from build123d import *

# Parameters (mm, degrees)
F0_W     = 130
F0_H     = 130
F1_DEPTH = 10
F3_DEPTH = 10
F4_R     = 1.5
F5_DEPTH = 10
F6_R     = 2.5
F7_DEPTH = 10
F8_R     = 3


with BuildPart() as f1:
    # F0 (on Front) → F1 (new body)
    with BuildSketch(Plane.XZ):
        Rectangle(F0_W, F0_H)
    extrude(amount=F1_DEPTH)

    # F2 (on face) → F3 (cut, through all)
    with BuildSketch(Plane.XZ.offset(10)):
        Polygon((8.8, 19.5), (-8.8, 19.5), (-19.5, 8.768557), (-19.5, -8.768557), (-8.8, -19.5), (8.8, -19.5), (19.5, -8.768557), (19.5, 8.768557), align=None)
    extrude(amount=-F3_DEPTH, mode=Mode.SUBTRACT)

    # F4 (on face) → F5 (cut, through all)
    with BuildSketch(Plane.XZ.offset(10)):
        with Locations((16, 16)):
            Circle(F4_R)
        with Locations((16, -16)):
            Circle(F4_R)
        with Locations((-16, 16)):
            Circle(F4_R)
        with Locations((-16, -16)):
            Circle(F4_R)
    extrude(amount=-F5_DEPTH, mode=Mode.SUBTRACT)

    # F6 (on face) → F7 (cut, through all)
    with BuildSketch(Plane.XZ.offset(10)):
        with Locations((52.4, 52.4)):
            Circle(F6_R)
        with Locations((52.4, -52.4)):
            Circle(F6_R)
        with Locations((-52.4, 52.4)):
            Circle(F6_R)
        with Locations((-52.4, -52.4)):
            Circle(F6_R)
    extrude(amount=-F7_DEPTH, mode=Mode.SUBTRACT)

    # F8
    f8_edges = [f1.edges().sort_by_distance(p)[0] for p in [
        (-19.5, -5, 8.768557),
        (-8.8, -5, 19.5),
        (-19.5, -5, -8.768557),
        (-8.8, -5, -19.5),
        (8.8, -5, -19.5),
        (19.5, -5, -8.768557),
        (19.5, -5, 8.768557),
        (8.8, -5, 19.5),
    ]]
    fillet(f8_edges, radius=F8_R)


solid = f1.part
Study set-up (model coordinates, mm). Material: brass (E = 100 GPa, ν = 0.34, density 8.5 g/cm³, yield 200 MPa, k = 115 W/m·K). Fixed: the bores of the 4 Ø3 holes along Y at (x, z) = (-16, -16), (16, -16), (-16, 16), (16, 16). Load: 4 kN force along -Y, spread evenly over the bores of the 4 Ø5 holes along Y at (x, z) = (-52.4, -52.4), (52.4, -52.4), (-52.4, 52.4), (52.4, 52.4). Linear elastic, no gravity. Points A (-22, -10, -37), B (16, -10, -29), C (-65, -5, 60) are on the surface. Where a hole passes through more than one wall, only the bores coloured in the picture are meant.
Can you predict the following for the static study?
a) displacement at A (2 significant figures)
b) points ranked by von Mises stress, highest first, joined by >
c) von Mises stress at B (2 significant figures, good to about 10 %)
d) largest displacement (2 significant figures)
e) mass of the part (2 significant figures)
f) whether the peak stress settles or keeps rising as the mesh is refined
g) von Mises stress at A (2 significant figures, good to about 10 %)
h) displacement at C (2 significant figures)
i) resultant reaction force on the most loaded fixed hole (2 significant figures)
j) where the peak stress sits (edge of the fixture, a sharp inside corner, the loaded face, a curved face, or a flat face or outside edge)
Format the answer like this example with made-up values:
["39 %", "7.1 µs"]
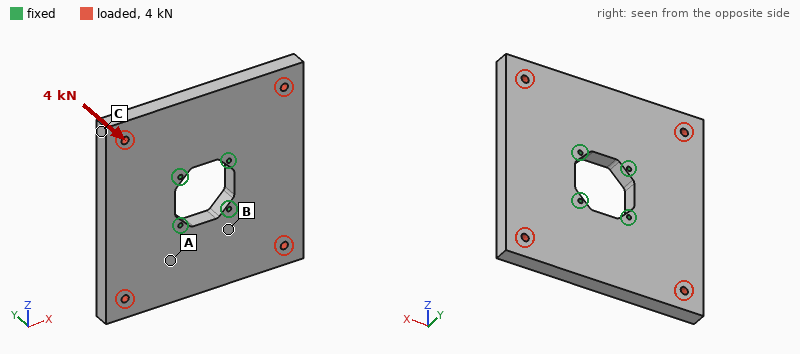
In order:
["0.032 mm", "B > A > C", "29 MPa", "0.15 mm", "1.3 kg", "keeps rising", "24 MPa", "0.14 mm", "1.0 kN", "edge of the fixture"]
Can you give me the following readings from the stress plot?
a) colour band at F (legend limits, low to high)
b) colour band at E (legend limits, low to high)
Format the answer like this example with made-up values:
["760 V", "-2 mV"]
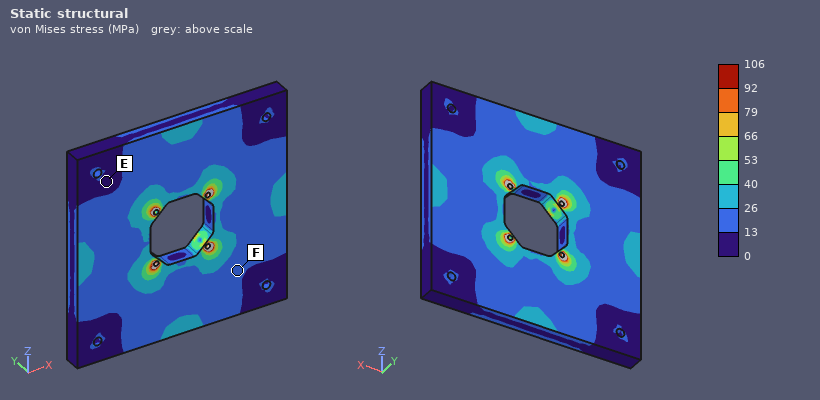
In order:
["13 to 26 MPa", "0 to 13 MPa"]
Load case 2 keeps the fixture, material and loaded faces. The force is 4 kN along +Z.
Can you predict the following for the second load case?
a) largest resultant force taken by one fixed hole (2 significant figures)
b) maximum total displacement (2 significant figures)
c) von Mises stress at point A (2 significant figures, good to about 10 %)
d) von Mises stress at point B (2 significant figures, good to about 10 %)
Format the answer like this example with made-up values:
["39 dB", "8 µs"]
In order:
["1.0 kN", "4.0 µm", "3.0 MPa", "3.3 MPa"]
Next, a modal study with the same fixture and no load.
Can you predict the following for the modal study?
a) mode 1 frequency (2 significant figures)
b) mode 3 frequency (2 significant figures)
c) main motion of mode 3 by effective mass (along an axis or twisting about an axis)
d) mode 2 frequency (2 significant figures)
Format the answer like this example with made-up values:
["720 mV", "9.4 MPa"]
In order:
["1400 Hz", "1500 Hz", "along Y", "1400 Hz"]
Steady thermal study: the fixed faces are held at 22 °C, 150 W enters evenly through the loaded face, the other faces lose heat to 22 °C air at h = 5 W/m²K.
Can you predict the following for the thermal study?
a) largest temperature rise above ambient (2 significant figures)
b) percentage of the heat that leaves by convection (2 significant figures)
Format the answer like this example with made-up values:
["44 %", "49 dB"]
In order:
["51 K", "3.4 %"]
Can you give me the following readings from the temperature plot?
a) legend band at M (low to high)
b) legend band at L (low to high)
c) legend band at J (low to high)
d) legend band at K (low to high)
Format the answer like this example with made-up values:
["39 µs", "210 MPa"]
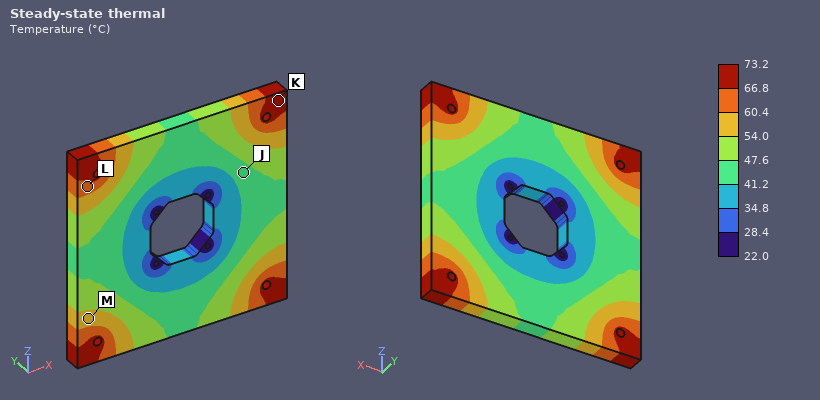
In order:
["54.0 to 60.4 °C", "60.4 to 66.8 °C", "41.2 to 47.6 °C", "66.8 to 73.2 °C"]
